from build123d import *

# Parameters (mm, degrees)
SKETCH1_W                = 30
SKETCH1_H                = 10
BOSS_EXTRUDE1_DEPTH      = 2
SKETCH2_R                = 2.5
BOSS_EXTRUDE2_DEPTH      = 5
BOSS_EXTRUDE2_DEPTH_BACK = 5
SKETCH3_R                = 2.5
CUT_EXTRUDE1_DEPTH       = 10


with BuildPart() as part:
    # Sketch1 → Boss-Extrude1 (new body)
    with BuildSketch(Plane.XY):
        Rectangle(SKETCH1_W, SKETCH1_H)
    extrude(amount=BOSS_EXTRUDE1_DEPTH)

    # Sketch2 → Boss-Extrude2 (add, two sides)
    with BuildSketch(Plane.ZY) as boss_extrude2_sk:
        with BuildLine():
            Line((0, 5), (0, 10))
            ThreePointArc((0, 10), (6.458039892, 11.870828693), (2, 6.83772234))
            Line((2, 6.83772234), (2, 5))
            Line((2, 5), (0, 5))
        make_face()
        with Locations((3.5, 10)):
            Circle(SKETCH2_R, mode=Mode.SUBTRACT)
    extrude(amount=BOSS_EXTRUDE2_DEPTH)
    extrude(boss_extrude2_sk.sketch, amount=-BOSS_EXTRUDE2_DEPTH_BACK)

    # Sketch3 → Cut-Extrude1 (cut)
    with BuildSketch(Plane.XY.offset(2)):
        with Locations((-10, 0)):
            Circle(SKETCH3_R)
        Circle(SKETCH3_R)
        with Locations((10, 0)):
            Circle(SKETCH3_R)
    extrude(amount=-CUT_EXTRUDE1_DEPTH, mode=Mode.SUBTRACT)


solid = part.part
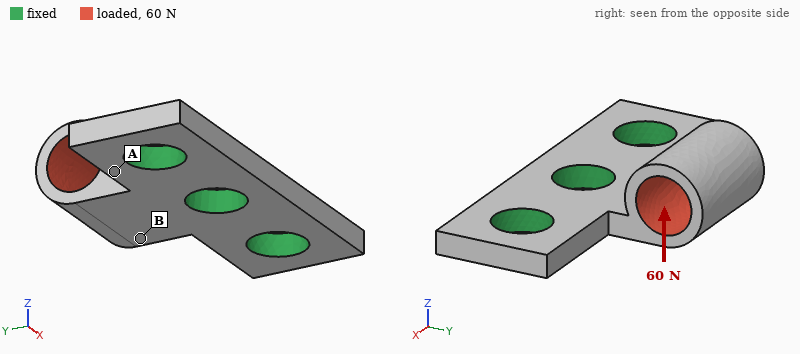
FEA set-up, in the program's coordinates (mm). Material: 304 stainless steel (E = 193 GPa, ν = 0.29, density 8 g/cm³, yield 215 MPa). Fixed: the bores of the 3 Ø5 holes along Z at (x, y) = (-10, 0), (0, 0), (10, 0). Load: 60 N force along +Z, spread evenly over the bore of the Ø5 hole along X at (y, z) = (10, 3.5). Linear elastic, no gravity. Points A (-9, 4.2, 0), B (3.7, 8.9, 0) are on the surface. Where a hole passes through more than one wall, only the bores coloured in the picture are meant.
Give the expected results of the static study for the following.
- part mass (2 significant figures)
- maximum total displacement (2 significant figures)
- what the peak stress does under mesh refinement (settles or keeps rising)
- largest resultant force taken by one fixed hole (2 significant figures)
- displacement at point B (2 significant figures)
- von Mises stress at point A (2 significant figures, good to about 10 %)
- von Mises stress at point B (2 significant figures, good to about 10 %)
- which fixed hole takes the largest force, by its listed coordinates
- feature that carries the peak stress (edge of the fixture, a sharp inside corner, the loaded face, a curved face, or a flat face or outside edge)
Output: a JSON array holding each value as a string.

["5.8 g", "14 µm", "keeps rising", "55 N", "5.8 µm", "10 MPa", "23 MPa", "(0, 0)", "edge of the fixture"]
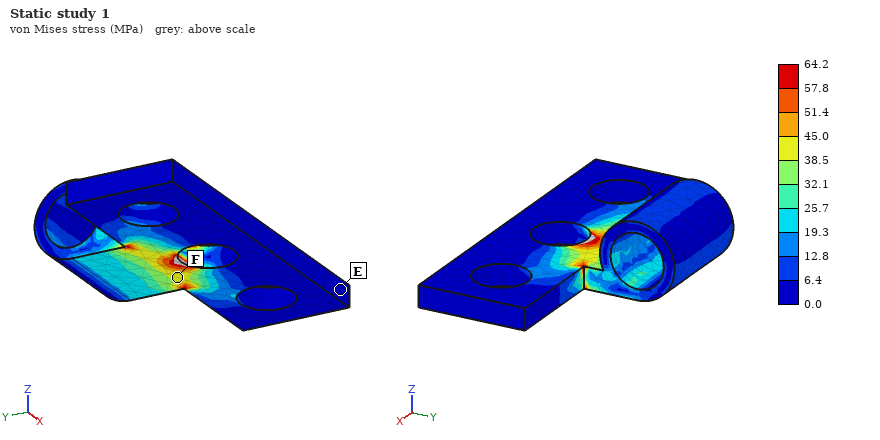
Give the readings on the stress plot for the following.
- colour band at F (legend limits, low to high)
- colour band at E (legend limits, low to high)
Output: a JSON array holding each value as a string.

["38.5 to 45.0 MPa", "0.0 to 6.4 MPa"]
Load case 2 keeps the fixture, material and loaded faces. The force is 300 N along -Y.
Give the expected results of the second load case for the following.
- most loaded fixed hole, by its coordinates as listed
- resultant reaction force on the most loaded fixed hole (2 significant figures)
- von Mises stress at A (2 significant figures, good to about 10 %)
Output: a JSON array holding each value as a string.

["(0, 0)", "240 N", "15 MPa"]
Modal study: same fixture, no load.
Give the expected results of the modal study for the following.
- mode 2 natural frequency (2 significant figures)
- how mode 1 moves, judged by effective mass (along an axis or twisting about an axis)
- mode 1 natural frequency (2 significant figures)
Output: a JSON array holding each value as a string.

["21 kHz", "along Z", "8800 Hz"]
